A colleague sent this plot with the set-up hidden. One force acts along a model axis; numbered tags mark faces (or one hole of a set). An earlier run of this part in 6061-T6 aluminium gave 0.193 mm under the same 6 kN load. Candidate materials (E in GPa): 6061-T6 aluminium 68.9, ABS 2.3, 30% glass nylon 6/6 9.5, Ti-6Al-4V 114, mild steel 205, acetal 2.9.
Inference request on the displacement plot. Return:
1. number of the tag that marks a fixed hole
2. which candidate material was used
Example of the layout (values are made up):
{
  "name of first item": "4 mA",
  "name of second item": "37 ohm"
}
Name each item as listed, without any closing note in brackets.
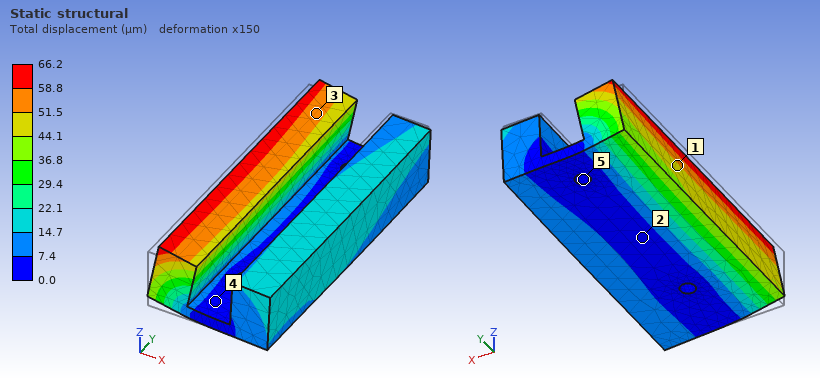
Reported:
{
  "number of the tag that marks a fixed hole": "5",
  "which candidate material was used": "mild steel"
}
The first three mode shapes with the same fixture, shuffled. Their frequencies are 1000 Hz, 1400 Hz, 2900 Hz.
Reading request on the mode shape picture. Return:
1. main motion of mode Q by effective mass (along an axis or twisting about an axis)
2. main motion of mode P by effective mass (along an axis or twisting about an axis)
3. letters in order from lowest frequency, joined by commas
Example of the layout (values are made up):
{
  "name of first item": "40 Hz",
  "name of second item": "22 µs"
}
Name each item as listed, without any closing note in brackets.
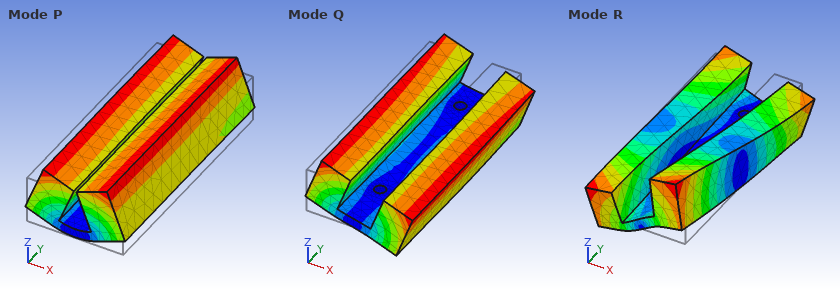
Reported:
{
  "main motion of mode Q by effective mass": "along X",
  "main motion of mode P by effective mass": "along Z",
  "letters in order from lowest frequency, joined by commas": "Q, P, R"
}
